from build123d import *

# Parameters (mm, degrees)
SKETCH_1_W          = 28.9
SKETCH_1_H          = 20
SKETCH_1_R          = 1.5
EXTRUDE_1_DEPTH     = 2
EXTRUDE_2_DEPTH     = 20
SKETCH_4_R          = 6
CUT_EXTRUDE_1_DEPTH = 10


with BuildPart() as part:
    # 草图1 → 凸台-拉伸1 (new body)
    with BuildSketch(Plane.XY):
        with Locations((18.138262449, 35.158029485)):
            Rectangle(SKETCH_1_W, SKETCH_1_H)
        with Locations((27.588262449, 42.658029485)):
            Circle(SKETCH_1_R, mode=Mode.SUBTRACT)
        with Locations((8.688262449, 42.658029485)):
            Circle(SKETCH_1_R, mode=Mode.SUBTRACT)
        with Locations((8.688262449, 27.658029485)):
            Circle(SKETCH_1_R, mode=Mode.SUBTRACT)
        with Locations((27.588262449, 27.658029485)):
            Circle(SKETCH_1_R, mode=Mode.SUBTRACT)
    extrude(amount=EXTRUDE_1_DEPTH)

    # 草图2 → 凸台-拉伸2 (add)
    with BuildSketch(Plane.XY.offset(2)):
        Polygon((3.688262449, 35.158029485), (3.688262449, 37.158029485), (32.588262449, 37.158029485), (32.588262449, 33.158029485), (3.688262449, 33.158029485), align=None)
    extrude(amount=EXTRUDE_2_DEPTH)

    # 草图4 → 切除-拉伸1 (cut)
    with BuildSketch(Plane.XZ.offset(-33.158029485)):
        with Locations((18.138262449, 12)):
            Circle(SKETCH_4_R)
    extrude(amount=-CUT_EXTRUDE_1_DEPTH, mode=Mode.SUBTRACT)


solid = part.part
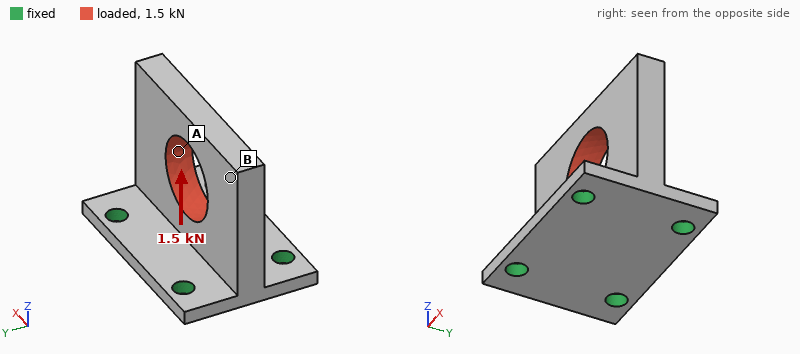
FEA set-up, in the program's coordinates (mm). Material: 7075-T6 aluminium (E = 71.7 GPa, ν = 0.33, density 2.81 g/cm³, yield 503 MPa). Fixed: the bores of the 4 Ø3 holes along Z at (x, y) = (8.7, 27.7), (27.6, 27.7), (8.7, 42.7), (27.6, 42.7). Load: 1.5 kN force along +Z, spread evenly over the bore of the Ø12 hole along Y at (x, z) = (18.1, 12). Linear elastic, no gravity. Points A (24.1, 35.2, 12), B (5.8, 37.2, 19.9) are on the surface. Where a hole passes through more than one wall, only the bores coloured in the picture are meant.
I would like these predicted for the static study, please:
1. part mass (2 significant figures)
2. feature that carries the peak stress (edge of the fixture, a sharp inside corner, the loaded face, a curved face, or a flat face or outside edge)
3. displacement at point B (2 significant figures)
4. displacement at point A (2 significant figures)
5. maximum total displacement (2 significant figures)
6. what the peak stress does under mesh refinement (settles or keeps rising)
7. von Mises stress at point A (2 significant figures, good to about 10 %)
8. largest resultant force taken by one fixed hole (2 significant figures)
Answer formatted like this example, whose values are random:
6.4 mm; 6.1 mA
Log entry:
8.3 g; edge of the fixture; 17 µm; 19 µm; 23 µm; keeps rising; 39 MPa; 390 N
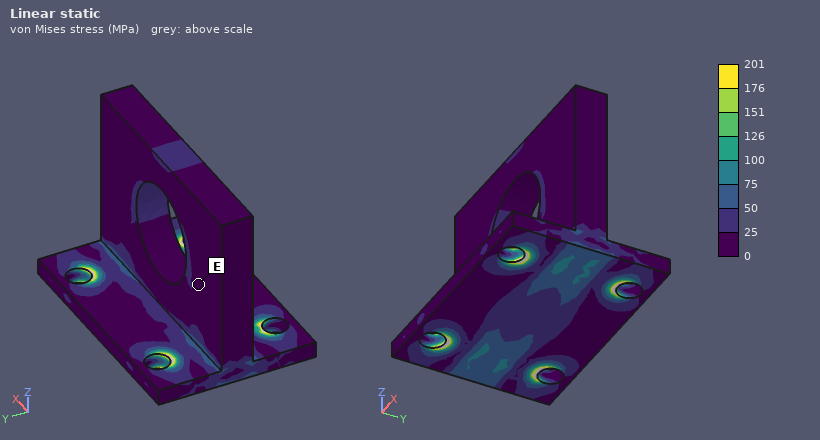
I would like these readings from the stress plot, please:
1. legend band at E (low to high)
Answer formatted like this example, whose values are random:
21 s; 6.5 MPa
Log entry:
0 to 25 MPa
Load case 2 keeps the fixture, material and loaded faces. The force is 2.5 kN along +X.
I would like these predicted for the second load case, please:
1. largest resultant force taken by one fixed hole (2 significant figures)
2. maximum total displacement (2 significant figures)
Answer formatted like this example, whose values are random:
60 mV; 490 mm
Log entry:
970 N; 0.13 mm
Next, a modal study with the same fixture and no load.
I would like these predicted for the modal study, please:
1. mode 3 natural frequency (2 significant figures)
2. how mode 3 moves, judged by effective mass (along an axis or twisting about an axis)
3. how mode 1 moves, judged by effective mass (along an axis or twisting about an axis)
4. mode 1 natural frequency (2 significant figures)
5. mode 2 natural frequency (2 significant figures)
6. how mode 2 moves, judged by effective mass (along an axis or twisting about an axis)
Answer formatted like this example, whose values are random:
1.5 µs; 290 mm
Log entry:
11 kHz; along X; along Y; 5500 Hz; 10 kHz; twisting about Z
